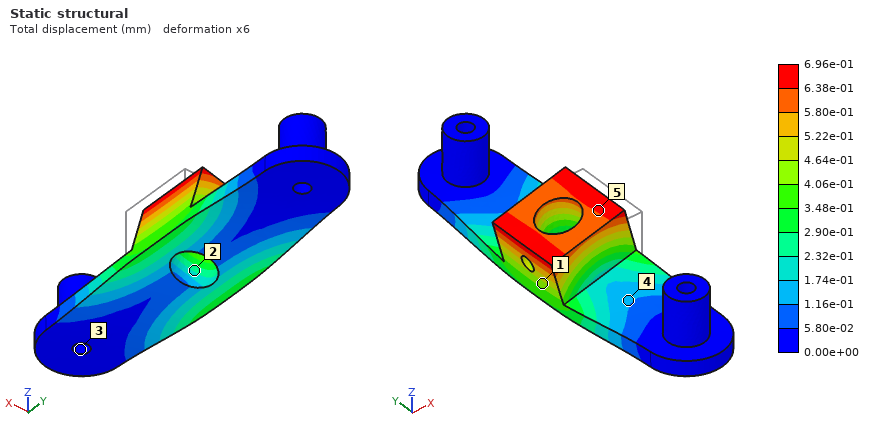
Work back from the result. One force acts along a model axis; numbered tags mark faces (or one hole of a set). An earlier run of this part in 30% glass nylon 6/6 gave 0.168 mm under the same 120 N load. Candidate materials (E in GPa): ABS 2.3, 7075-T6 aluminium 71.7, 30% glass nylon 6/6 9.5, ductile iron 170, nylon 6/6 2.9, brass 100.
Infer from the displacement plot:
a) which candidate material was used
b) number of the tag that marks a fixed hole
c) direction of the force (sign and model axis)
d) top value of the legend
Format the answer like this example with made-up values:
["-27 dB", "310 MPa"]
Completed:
["ABS", "3", "-X", "6.96e-01 mm"]
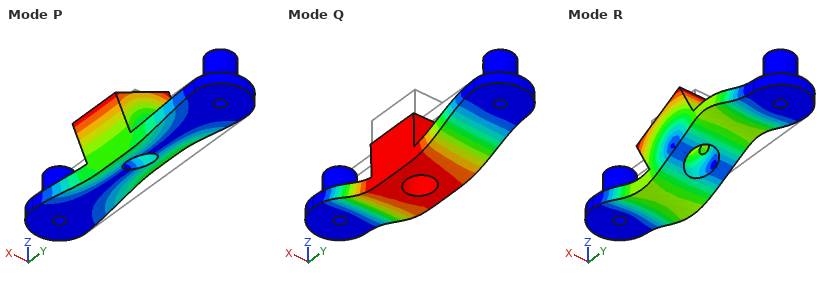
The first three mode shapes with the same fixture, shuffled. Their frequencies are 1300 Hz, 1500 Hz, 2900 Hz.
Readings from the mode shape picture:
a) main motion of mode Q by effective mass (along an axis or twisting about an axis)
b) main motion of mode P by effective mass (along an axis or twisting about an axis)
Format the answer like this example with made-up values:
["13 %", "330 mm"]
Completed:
["along Z", "along X"]
